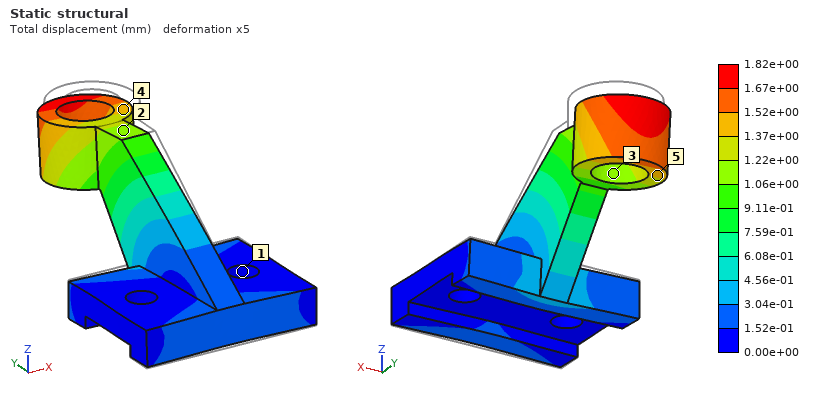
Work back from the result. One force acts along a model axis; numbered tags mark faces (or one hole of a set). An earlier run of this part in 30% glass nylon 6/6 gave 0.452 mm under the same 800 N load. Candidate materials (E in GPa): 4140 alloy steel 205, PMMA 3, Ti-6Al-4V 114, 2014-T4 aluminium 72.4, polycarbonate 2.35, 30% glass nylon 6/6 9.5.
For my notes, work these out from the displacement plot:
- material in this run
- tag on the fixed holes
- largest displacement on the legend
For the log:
polycarbonate
1
1.82e+00 mm
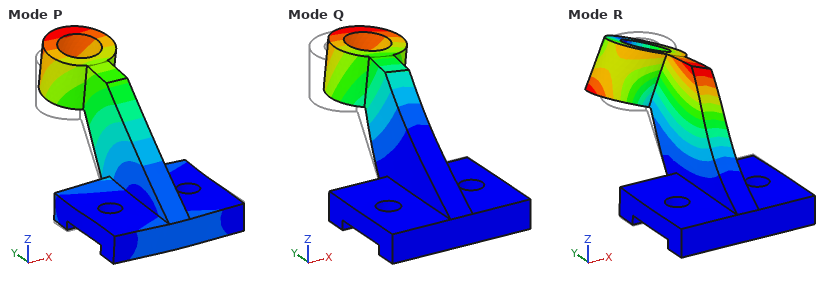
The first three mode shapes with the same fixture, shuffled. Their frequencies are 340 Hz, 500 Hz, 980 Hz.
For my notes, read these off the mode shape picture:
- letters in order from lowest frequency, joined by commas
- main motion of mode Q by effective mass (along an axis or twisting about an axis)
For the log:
Q, P, R
along X
